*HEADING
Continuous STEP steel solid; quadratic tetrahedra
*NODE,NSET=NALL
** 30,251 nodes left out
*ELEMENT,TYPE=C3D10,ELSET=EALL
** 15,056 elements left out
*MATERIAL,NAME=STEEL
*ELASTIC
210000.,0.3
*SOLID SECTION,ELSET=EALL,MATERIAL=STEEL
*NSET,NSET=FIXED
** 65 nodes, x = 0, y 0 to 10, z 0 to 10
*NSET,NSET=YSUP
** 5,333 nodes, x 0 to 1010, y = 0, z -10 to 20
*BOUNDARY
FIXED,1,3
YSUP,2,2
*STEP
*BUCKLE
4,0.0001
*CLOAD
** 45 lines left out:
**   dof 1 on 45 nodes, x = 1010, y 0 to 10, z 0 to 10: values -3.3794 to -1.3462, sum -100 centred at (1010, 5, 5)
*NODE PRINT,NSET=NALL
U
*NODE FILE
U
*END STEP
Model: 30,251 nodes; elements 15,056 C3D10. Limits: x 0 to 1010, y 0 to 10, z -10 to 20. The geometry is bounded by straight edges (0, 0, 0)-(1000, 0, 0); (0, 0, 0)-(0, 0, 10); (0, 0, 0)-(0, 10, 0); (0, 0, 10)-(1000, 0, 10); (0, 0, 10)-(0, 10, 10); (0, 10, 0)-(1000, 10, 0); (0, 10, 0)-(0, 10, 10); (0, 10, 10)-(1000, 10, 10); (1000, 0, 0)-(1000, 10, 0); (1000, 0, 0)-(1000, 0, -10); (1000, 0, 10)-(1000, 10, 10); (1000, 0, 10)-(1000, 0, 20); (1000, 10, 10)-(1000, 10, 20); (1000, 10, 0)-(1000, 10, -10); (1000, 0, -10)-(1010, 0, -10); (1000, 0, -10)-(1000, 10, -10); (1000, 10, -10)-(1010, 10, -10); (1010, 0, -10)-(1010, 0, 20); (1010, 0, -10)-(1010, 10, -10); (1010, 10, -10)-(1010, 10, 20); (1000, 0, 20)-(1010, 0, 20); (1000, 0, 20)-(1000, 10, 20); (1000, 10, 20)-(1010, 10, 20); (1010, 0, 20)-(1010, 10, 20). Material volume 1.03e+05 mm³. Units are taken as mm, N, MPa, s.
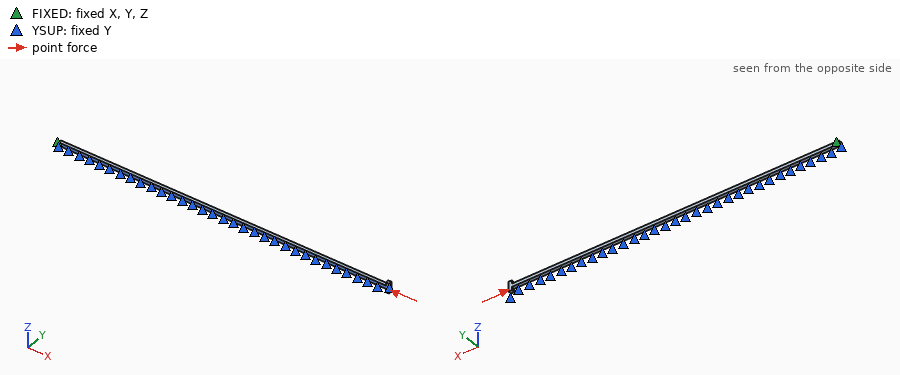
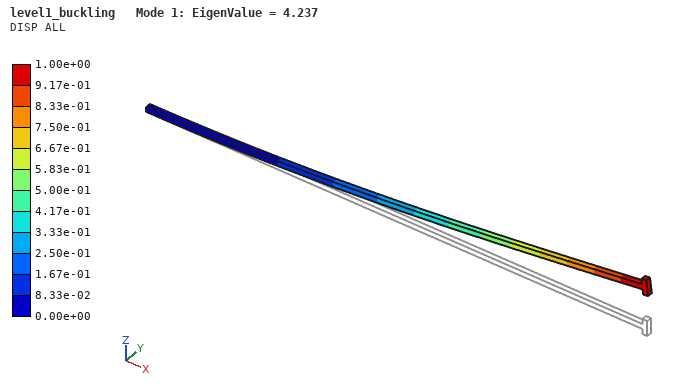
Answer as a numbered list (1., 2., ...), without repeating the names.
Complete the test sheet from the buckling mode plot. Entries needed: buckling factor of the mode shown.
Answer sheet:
1. 4.237
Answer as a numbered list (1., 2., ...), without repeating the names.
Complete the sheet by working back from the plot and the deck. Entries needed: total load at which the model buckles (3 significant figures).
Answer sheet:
1. 424 N
